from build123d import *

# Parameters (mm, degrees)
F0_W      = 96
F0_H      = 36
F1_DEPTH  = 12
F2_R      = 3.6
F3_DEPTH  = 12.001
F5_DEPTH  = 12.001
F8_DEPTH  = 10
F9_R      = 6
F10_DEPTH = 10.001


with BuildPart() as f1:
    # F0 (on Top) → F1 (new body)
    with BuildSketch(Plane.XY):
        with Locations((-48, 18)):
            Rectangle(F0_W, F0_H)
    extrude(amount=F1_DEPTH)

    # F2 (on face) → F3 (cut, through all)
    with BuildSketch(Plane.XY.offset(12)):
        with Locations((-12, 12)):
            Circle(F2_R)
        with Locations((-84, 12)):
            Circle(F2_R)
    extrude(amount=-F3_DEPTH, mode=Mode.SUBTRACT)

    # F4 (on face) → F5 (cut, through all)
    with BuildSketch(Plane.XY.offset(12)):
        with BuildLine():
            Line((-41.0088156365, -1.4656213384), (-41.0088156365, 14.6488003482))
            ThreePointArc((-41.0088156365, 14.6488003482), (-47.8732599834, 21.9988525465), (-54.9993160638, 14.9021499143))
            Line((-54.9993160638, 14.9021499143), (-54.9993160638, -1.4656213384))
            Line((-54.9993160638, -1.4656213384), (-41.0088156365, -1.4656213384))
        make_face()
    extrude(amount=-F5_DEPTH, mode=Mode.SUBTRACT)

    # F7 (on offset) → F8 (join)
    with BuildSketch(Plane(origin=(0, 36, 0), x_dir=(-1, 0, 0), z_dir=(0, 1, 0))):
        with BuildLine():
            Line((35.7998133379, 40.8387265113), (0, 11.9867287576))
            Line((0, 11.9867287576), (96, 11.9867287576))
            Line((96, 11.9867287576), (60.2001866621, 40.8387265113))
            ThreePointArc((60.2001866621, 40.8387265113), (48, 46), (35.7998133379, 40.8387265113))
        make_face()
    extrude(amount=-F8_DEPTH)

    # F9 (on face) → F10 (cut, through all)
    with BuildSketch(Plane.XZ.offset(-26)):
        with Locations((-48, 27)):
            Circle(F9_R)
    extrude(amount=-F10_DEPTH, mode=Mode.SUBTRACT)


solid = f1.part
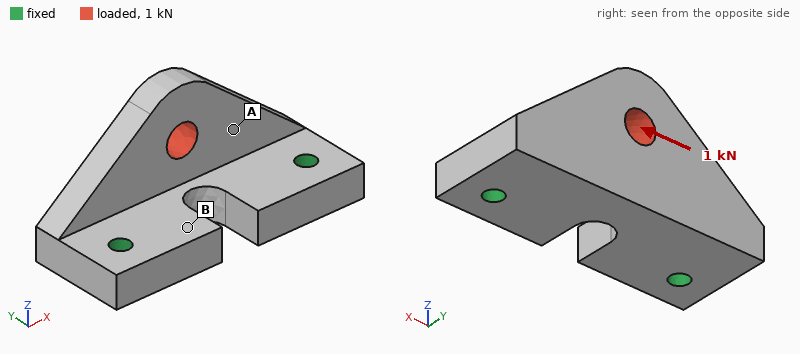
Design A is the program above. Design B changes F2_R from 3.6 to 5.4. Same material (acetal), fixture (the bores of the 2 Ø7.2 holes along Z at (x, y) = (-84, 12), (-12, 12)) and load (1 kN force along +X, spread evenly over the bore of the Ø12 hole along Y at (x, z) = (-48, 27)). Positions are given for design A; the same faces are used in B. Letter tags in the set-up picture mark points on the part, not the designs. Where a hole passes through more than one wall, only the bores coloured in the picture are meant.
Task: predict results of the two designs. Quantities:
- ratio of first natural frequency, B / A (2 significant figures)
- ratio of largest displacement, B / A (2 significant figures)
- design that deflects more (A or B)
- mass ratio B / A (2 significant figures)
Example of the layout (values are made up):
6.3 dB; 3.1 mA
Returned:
1.1; 0.83; A; 0.98
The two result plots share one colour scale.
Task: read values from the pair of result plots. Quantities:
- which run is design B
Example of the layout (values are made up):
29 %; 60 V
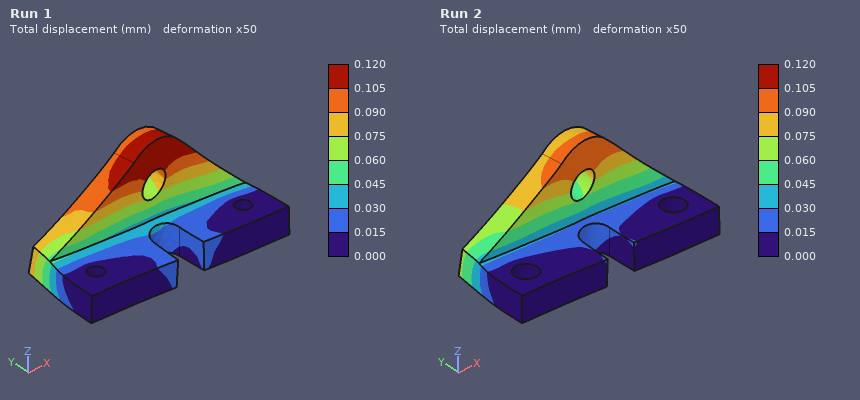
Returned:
Run 2
